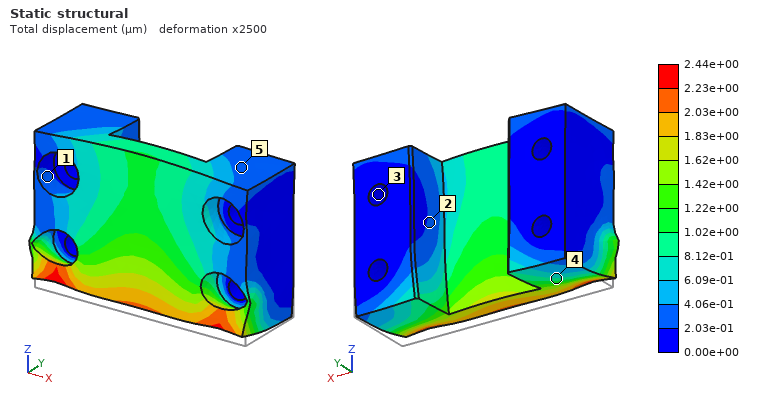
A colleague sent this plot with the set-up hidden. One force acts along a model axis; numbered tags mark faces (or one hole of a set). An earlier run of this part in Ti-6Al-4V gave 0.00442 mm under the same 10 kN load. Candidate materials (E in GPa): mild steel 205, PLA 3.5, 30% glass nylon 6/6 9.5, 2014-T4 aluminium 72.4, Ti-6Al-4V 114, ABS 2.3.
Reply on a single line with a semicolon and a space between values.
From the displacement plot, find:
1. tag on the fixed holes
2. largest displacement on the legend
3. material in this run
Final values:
3; 2.44e+00 µm; mild steel
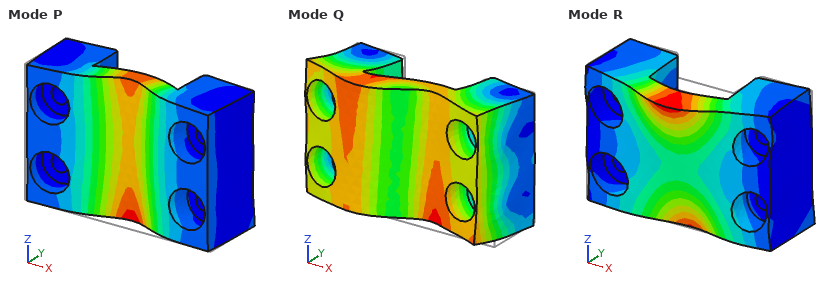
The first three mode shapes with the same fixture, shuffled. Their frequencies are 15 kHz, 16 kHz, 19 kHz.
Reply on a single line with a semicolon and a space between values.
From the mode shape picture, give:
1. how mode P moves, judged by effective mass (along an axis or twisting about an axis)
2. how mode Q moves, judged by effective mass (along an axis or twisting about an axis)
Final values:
along Y; along X
